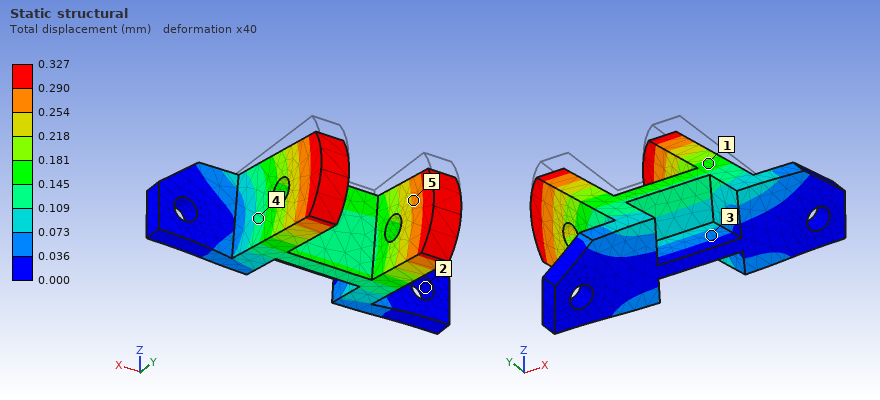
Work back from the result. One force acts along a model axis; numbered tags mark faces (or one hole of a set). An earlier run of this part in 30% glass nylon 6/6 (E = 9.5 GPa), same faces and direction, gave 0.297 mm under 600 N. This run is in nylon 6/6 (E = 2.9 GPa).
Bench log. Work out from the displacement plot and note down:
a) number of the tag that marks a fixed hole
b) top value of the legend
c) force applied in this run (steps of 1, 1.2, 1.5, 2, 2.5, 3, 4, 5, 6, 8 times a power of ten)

2
0.327 mm
200 N
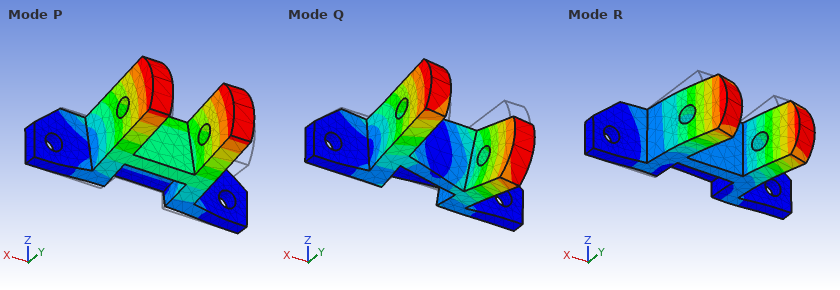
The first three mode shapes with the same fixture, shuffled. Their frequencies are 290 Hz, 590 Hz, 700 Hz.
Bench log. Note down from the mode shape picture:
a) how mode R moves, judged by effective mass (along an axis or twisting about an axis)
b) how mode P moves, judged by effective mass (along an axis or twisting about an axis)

along X
along Z
